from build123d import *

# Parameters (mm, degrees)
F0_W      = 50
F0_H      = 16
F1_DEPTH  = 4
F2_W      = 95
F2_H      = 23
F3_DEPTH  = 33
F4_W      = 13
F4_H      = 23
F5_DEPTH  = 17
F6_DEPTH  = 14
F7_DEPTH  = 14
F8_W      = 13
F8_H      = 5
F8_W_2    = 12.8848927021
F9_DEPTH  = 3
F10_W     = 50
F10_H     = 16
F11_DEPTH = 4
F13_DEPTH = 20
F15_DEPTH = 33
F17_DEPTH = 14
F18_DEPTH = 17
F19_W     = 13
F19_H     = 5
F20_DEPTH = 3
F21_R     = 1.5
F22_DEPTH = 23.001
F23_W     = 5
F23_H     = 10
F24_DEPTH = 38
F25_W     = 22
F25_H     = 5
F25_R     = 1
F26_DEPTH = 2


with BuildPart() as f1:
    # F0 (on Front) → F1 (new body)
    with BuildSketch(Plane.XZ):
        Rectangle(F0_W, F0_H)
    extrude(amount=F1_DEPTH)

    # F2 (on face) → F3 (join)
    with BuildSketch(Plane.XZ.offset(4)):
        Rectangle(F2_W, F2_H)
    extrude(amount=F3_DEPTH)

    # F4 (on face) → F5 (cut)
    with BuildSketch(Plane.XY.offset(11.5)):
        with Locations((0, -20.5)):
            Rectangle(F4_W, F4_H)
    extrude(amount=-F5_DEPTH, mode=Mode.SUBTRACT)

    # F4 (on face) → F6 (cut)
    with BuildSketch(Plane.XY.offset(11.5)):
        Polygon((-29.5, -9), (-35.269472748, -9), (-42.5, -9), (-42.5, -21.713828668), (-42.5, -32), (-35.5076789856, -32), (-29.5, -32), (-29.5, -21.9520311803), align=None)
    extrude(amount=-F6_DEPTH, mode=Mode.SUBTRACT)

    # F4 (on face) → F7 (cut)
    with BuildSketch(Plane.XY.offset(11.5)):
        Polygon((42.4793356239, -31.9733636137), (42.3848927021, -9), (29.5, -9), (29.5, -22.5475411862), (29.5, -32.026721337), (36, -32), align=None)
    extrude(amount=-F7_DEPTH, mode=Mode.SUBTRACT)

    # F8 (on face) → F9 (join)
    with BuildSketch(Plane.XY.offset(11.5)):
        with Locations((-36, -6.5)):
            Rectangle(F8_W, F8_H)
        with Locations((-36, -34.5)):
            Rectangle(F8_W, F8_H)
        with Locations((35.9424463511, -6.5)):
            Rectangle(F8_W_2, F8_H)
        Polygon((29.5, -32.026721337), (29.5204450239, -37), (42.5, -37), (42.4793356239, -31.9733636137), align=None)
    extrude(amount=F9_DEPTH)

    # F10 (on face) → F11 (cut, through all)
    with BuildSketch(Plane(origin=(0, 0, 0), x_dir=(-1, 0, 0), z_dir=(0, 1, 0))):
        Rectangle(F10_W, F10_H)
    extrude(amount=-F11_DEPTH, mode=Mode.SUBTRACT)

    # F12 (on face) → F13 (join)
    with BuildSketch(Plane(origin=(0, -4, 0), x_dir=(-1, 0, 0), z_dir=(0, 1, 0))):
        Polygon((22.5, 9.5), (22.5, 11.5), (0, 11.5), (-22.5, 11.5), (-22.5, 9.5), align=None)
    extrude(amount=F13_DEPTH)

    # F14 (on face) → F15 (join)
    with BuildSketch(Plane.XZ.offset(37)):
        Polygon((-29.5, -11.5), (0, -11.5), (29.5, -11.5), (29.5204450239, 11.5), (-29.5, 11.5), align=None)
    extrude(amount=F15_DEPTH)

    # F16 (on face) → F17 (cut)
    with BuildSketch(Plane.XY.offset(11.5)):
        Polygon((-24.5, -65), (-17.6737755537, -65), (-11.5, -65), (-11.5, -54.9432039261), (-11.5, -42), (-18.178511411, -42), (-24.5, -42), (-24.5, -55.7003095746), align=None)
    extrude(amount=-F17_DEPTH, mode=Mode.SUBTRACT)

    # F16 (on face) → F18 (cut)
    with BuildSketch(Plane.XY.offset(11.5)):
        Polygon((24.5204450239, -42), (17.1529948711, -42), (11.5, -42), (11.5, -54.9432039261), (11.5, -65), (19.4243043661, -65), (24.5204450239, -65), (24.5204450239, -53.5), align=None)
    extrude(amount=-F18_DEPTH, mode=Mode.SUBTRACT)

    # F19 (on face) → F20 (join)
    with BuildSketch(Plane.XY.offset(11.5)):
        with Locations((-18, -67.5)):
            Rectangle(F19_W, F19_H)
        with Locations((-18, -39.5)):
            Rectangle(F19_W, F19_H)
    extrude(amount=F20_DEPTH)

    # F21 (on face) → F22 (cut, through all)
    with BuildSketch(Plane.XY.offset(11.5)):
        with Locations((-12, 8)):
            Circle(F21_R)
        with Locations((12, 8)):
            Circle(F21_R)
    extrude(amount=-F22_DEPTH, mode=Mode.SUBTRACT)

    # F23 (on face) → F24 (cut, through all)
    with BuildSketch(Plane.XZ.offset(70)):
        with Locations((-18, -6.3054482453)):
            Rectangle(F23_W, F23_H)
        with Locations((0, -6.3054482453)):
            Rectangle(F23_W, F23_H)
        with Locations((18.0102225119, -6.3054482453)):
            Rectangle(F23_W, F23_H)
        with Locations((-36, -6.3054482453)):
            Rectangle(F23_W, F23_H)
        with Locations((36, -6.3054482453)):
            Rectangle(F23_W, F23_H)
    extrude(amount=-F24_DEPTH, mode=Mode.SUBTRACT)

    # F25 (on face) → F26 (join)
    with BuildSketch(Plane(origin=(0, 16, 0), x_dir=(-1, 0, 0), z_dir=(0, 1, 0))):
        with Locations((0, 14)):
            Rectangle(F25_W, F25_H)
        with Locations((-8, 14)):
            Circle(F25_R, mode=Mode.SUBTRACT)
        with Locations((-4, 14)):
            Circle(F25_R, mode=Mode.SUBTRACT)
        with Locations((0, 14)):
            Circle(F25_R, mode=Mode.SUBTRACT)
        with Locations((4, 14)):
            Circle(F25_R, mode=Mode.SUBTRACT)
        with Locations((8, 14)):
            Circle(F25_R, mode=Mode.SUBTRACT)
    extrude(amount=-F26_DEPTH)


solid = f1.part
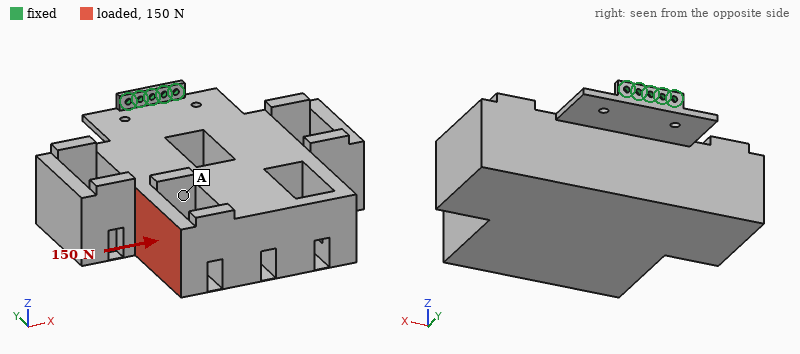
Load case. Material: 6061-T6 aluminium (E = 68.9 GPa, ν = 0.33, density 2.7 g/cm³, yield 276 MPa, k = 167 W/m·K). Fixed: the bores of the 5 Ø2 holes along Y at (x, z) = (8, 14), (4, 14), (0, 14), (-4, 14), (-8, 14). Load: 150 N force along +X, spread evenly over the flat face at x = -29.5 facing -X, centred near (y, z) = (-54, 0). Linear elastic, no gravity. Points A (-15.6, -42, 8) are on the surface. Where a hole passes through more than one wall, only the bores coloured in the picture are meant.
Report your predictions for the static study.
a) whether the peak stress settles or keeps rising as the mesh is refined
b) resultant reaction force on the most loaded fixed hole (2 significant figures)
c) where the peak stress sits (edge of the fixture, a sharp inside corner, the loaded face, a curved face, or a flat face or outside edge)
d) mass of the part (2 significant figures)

keeps rising
510 N
edge of the fixture
250 g
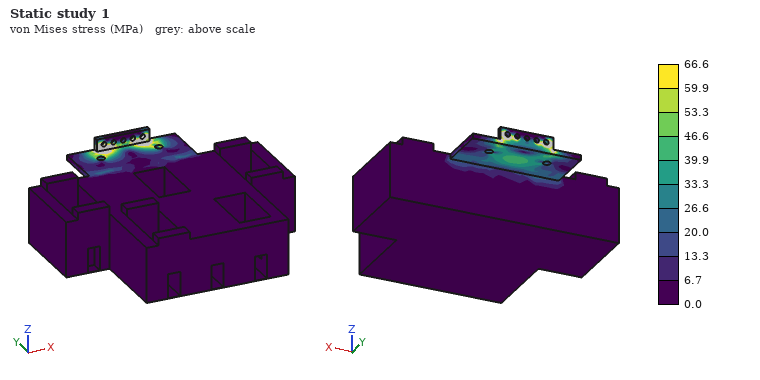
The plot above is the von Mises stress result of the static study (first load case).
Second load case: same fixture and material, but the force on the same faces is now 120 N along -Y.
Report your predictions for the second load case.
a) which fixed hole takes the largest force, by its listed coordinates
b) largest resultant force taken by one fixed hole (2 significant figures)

(-8, 14)
190 N
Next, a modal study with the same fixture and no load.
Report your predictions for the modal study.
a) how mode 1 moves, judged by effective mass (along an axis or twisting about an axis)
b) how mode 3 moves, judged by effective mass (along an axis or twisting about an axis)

along Z
along X
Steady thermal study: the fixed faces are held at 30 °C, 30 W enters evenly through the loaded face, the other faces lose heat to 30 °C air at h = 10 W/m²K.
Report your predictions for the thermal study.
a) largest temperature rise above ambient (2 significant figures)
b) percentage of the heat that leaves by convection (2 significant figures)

57 K
38 %
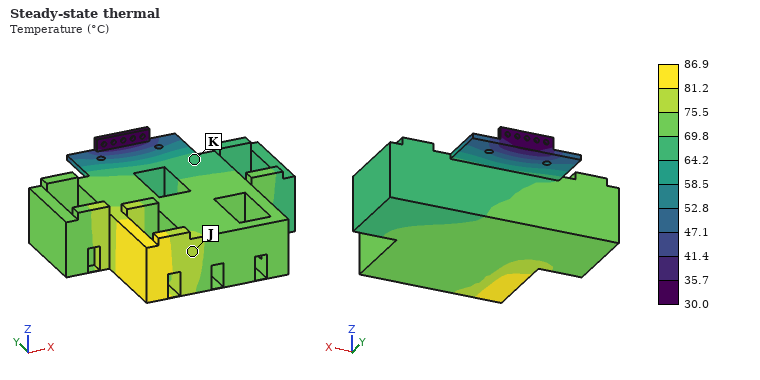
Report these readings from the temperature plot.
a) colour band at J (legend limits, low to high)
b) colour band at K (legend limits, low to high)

75.5 to 81.2 °C
64.2 to 69.8 °C
